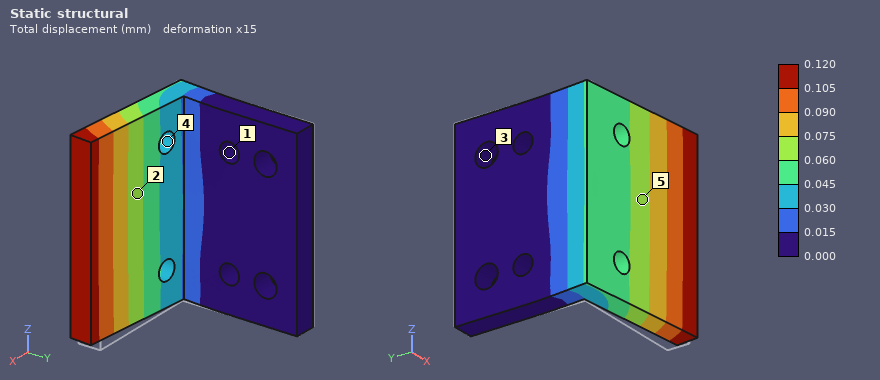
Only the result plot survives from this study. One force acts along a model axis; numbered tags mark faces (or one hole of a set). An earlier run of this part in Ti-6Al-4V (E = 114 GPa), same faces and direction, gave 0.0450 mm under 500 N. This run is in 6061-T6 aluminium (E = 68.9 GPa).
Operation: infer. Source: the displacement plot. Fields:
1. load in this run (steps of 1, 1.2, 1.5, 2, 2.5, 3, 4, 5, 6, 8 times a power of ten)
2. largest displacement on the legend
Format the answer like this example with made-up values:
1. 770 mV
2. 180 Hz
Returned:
1. 800 N
2. 0.120 mm
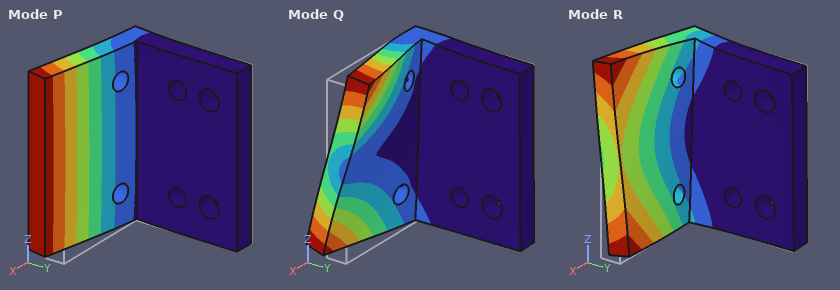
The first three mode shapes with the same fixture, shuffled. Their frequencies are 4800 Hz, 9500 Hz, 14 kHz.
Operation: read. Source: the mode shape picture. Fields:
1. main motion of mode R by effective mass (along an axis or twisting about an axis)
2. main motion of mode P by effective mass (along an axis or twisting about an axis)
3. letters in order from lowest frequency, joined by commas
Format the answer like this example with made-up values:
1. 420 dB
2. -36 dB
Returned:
1. along Z
2. along Y
3. P, R, Q
